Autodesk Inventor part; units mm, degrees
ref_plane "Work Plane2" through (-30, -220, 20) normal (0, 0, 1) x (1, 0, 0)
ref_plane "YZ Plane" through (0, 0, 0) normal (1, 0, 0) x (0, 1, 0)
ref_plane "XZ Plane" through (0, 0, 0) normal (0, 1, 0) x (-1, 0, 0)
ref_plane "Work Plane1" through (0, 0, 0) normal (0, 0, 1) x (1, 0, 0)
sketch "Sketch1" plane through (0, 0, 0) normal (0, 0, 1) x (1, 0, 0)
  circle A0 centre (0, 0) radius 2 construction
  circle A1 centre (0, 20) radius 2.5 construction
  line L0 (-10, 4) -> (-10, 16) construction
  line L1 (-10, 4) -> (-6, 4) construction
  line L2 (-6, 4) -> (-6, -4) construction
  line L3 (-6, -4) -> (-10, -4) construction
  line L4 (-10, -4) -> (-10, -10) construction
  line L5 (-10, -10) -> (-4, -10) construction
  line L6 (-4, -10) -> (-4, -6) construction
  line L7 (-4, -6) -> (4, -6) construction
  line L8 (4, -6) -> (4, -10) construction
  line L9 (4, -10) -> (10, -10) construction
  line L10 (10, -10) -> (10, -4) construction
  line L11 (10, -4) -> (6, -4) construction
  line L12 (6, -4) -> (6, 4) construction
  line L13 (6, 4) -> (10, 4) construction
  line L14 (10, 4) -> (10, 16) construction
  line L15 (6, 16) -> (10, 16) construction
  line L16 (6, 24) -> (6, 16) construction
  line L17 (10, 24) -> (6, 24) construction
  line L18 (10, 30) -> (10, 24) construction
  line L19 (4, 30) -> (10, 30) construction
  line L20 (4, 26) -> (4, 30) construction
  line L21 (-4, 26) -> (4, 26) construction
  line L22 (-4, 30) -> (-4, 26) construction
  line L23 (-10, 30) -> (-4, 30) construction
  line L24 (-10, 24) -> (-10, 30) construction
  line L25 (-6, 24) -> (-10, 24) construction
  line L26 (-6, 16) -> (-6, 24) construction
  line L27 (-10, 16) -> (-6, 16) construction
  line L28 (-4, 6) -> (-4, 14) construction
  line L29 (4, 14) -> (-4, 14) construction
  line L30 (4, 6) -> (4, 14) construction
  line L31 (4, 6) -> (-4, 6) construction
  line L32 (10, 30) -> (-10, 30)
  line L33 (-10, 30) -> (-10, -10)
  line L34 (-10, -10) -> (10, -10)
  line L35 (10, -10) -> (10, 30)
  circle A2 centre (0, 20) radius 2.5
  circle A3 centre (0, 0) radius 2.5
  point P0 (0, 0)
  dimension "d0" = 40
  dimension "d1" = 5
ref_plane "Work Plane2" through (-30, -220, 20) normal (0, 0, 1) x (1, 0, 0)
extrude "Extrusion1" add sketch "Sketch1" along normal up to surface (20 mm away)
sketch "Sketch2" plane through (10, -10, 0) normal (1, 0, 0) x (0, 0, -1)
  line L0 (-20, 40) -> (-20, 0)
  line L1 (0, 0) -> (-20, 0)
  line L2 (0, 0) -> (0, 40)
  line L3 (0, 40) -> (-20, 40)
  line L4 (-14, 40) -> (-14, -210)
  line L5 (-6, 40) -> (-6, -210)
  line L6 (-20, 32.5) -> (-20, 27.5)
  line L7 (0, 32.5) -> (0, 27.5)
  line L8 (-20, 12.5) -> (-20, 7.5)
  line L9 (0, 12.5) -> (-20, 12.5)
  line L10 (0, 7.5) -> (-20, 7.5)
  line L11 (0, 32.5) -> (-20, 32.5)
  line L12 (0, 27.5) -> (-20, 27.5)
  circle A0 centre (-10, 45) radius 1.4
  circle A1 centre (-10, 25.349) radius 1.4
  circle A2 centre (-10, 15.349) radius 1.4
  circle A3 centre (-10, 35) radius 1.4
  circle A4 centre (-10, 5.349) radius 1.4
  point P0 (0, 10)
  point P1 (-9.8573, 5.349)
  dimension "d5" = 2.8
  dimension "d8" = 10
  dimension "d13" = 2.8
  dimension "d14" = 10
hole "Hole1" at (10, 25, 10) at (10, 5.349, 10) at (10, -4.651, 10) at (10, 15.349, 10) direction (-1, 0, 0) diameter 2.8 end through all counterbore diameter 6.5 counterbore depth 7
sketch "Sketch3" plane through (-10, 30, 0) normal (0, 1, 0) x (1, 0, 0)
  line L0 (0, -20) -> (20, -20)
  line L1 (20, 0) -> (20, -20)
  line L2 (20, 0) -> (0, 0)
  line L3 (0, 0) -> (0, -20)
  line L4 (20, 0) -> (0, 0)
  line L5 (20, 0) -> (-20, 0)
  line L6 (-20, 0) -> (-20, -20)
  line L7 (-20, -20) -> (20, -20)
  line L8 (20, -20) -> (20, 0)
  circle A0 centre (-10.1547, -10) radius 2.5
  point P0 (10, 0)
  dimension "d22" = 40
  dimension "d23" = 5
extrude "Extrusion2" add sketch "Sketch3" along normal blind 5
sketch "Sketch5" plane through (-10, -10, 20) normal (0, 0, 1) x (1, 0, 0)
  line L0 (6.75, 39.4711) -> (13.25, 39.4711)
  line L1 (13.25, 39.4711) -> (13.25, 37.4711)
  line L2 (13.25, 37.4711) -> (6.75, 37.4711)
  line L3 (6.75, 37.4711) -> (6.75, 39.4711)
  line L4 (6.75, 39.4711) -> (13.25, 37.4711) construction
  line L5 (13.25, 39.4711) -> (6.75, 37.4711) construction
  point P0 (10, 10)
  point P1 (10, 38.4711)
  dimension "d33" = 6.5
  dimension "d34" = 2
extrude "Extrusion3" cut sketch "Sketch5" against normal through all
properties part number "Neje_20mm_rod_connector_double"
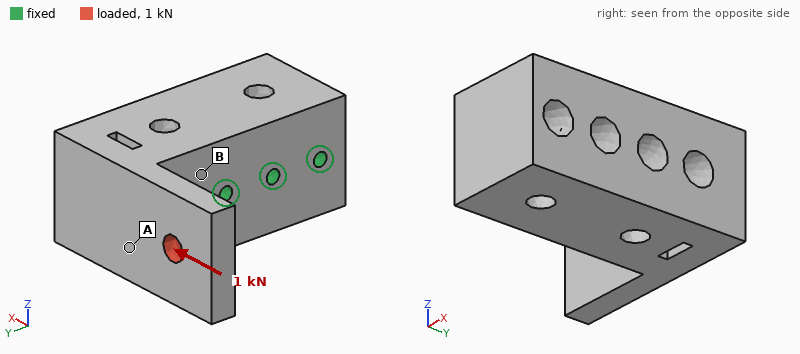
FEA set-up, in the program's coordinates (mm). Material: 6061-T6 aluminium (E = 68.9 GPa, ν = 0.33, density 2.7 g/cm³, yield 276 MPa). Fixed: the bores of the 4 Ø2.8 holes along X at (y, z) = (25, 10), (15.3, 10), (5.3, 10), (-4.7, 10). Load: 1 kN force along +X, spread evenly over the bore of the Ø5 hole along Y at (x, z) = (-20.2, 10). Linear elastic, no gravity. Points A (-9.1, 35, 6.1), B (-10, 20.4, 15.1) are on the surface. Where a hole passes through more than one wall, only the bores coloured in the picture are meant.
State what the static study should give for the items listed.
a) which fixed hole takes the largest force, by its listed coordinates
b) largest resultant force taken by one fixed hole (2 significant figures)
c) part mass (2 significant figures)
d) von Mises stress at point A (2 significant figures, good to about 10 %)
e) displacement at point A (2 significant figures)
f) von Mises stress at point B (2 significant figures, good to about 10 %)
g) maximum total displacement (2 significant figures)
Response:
(25, 10)
1.1 kN
48 g
12 MPa
4.7 µm
5.5 MPa
12 µm
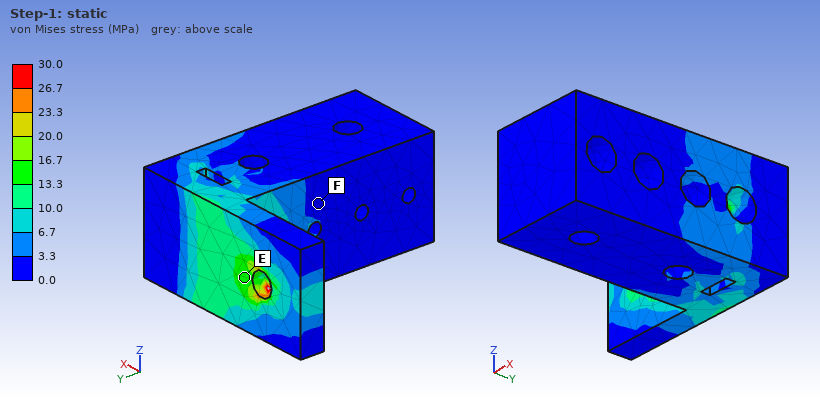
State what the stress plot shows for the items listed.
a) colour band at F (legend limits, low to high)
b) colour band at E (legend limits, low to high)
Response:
0.0 to 3.3 MPa
13.3 to 16.7 MPa
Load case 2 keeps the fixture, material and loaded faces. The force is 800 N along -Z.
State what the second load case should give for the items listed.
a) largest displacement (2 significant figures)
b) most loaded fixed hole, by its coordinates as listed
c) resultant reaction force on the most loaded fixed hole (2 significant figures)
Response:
28 µm
(25, 10)
1.1 kN
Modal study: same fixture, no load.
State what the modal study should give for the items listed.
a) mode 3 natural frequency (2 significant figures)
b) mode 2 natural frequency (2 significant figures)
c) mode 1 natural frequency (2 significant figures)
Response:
17 kHz
13 kHz
7500 Hz
